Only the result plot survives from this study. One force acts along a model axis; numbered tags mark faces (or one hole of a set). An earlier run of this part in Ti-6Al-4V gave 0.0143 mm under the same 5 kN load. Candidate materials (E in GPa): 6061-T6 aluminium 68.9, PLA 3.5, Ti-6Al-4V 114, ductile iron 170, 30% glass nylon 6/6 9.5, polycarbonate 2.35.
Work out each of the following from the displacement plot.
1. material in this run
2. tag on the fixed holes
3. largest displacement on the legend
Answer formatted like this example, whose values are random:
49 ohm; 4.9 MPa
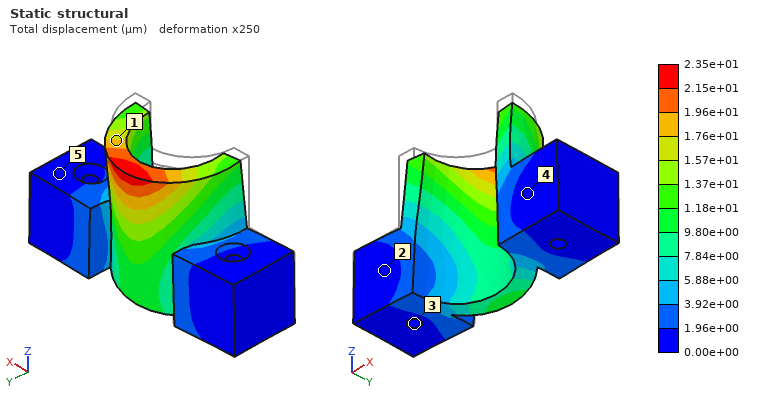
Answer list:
6061-T6 aluminium; 3; 2.35e+01 µm
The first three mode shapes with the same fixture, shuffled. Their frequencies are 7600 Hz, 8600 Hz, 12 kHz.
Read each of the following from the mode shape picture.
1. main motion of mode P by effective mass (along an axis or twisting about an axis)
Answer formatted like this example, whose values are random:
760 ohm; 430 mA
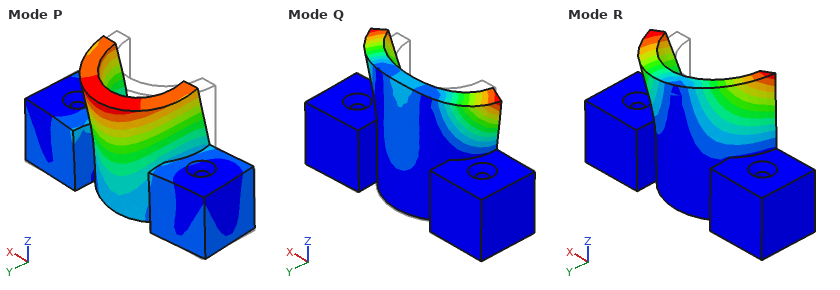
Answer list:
along Y
